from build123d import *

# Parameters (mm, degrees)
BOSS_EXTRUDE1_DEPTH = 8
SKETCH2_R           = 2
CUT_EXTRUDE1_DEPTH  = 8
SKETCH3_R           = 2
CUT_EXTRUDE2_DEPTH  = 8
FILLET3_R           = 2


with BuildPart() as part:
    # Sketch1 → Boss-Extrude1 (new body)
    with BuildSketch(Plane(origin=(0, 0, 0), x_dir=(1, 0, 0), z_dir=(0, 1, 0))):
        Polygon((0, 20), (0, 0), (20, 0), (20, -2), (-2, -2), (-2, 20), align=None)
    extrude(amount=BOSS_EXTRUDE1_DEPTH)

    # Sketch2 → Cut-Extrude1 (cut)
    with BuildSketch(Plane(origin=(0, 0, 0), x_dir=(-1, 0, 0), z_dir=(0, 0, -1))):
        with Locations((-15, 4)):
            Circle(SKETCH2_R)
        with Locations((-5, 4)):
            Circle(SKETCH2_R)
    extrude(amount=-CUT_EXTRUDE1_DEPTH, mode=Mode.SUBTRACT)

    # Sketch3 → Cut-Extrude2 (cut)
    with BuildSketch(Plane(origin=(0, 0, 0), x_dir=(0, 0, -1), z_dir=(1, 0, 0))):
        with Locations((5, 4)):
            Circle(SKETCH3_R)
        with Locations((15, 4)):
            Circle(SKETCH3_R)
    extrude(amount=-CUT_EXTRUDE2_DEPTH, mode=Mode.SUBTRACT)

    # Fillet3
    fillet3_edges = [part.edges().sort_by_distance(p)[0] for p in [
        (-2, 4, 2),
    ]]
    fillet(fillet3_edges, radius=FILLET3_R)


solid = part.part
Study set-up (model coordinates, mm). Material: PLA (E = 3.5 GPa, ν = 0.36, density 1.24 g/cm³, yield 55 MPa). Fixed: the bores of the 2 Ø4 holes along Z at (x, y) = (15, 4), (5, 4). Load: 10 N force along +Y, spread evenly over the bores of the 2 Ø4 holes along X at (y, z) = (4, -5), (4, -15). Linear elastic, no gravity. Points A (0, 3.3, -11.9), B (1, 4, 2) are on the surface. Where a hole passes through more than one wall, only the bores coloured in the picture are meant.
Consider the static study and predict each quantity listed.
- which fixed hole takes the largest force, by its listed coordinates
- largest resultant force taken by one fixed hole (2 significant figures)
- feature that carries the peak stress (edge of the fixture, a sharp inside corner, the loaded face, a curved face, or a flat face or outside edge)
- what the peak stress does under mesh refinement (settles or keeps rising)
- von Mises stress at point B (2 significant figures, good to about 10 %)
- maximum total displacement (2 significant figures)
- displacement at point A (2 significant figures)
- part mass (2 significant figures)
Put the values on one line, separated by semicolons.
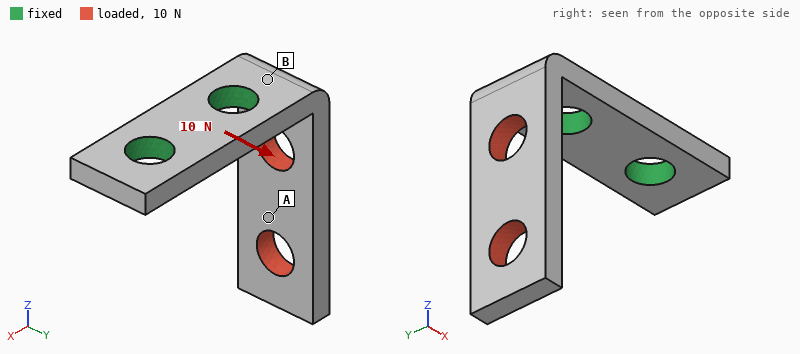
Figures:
(5, 4); 11 N; edge of the fixture; keeps rising; 11 MPa; 0.35 mm; 0.21 mm; 0.70 g
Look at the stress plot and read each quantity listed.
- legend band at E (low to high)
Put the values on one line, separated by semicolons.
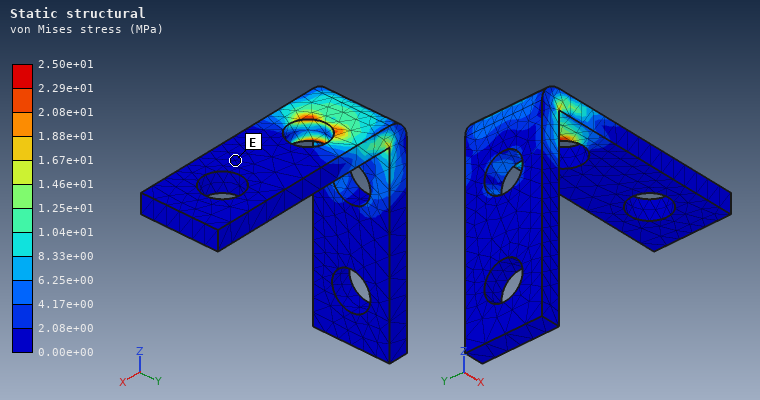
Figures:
0.00e+00 to 2.08e+00 MPa
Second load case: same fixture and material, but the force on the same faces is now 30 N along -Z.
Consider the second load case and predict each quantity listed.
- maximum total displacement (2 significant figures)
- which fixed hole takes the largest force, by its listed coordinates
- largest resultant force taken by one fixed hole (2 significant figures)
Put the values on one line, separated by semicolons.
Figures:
0.36 mm; (5, 4); 30 N
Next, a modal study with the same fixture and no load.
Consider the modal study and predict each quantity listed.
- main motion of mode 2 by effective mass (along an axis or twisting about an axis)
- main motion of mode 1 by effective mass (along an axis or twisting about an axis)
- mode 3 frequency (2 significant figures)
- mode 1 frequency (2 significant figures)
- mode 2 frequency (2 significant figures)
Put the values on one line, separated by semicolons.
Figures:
along Y; along X; 5000 Hz; 930 Hz; 1800 Hz
